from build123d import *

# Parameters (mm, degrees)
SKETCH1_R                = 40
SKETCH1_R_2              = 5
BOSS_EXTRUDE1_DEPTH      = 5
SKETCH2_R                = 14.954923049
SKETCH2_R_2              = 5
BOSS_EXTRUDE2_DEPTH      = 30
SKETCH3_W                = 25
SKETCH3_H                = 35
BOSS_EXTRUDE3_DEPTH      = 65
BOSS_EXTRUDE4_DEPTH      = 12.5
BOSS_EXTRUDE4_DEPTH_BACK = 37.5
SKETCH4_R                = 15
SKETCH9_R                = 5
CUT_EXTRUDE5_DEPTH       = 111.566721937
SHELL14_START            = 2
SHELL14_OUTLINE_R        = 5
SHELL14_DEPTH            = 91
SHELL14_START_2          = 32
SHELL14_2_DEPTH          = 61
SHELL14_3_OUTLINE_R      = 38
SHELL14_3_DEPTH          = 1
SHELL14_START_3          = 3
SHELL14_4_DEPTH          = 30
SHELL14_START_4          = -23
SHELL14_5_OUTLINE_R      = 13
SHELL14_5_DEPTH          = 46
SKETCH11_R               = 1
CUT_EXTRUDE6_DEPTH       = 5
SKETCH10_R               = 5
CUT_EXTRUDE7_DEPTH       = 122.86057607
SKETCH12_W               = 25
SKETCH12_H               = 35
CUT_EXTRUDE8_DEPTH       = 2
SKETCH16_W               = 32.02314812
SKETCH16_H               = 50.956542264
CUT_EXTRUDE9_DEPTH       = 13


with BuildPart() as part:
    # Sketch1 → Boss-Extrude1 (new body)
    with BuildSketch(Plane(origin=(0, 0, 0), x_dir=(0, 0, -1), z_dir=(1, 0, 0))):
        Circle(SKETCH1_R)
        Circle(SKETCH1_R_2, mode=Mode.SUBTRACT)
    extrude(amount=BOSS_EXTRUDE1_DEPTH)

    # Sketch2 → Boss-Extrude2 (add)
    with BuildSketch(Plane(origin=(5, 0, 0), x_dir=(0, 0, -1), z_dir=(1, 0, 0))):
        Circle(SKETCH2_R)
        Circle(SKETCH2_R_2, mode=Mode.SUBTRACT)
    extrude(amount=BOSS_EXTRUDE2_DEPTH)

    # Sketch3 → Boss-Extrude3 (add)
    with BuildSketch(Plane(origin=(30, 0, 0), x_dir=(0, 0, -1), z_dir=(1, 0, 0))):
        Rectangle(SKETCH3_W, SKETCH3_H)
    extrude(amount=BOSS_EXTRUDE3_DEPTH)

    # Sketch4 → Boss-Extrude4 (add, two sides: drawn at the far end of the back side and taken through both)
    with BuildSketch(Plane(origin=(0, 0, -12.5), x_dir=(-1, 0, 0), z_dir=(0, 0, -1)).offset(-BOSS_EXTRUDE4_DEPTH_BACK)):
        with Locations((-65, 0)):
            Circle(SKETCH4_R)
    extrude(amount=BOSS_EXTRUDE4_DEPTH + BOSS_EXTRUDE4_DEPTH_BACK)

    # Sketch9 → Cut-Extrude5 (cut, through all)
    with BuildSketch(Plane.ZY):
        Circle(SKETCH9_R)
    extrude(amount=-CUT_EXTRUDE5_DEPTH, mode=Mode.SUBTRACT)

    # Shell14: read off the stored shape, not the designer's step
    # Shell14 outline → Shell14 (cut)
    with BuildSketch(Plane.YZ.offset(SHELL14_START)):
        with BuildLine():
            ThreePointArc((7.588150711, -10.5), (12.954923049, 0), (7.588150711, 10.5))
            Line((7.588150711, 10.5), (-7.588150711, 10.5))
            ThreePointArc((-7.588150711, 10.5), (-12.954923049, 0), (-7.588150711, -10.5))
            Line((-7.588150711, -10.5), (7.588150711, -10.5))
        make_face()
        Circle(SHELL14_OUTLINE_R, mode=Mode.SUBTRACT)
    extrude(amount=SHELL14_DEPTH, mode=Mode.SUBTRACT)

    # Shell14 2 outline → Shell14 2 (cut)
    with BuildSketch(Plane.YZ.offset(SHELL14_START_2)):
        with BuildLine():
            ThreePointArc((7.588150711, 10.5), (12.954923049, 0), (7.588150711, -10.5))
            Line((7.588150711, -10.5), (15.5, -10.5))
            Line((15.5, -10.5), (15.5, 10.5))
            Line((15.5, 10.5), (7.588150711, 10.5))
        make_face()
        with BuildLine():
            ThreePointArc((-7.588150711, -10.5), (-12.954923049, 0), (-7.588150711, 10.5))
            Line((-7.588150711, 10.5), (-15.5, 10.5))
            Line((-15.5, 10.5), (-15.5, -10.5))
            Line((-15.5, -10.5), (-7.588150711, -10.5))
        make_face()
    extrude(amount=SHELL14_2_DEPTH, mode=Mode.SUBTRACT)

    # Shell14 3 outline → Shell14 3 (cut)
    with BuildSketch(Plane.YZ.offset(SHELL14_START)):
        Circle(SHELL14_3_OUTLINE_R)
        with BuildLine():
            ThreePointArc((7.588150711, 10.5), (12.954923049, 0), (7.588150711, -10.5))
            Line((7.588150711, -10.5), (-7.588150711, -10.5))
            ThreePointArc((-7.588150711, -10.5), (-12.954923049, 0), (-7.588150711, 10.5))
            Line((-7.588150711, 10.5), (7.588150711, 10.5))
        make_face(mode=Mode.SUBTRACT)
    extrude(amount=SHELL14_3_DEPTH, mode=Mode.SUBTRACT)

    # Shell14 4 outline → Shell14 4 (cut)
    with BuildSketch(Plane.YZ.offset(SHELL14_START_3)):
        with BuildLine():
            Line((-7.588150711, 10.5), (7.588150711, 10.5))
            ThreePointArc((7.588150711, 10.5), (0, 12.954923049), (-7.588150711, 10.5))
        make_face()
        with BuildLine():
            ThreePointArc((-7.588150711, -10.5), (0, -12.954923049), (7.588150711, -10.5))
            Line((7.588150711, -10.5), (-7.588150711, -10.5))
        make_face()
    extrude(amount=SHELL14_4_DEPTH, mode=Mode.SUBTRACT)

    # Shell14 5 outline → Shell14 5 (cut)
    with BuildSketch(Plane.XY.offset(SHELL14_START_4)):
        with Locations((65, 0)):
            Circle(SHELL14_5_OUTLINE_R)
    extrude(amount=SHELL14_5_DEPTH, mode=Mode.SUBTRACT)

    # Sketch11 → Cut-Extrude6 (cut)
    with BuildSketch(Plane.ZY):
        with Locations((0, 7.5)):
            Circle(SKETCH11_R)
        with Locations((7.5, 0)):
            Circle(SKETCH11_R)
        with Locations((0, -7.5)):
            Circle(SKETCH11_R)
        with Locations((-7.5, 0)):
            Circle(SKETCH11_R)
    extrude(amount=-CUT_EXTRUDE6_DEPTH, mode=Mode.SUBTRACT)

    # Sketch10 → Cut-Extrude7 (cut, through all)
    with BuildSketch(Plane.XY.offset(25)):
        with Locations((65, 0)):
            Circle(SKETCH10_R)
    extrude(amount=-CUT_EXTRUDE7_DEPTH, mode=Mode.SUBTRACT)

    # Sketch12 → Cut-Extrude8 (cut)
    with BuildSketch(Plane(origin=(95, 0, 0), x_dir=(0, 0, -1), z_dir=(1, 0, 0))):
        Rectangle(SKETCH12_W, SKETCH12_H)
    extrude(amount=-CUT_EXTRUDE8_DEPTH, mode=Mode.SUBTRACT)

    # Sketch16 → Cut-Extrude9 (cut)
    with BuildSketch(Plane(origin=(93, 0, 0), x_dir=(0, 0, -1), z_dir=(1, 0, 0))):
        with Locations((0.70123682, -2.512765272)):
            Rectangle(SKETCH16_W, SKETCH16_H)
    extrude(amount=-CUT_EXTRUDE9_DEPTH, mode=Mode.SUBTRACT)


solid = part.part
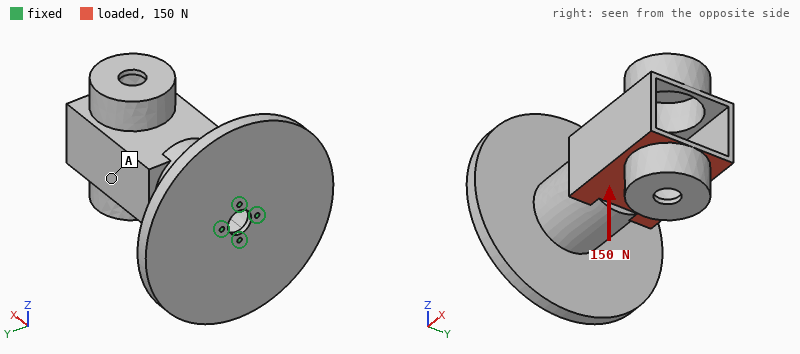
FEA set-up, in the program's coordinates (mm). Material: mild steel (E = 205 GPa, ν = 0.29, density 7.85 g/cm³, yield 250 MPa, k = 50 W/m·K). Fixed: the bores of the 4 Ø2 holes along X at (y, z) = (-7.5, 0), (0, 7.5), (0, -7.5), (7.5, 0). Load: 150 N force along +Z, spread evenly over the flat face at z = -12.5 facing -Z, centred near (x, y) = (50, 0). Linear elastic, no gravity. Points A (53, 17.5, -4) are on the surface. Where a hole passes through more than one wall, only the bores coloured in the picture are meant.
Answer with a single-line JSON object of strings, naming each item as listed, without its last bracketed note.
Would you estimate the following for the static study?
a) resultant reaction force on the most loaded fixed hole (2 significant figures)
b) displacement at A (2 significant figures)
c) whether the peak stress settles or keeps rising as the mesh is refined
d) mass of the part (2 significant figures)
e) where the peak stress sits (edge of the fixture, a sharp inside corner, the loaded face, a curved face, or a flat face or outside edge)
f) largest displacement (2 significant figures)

{"resultant reaction force on the most loaded fixed hole": "250 N", "displacement at A": "0.23 mm", "whether the peak stress settles or keeps rising as the mesh is refined": "keeps rising", "mass of the part": "310 g", "where the peak stress sits": "edge of the fixture", "largest displacement": "0.36 mm"}
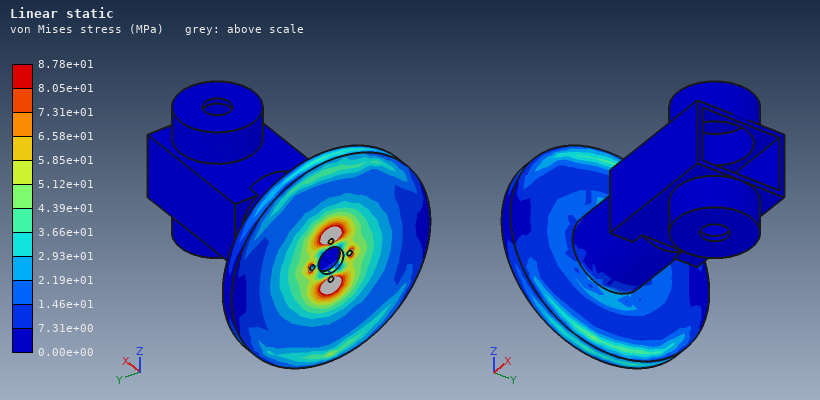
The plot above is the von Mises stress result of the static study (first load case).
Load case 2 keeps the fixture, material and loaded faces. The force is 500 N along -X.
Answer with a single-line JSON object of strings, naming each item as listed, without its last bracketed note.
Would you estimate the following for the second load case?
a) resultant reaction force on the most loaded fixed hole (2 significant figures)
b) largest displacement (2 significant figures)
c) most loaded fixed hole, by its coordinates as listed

{"resultant reaction force on the most loaded fixed hole": "340 N", "largest displacement": "0.36 mm", "most loaded fixed hole, by its coordinates as listed": "(0, -7.5)"}
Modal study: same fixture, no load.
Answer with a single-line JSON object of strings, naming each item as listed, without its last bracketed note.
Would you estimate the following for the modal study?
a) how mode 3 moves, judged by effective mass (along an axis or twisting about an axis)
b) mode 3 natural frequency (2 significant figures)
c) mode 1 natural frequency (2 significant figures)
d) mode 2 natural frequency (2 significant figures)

{"how mode 3 moves, judged by effective mass": "along X", "mode 3 natural frequency": "770 Hz", "mode 1 natural frequency": "290 Hz", "mode 2 natural frequency": "290 Hz"}
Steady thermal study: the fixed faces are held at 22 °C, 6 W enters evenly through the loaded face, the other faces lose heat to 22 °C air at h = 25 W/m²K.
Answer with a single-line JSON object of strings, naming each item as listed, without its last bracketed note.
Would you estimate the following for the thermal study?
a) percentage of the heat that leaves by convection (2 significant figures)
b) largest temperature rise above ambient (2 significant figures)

{"percentage of the heat that leaves by convection": "90 %", "largest temperature rise above ambient": "16 K"}
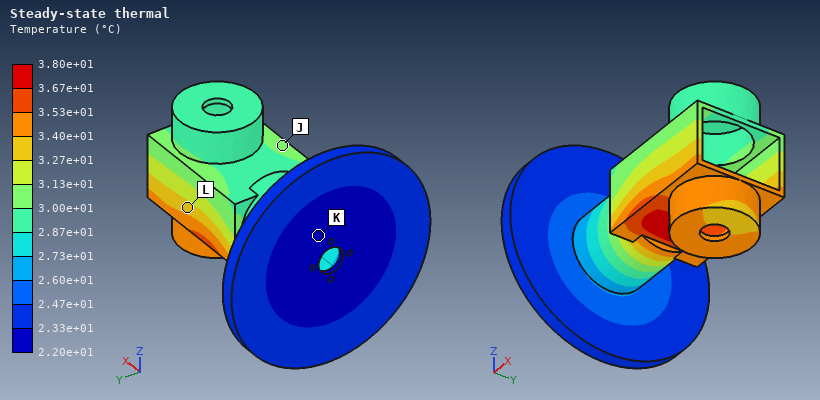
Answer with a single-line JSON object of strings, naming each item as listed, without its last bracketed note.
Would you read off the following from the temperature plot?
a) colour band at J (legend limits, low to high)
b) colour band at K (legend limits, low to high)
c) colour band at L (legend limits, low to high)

{"colour band at J": "3.00e+01 to 3.13e+01 °C", "colour band at K": "2.20e+01 to 2.33e+01 °C", "colour band at L": "3.27e+01 to 3.40e+01 °C"}
